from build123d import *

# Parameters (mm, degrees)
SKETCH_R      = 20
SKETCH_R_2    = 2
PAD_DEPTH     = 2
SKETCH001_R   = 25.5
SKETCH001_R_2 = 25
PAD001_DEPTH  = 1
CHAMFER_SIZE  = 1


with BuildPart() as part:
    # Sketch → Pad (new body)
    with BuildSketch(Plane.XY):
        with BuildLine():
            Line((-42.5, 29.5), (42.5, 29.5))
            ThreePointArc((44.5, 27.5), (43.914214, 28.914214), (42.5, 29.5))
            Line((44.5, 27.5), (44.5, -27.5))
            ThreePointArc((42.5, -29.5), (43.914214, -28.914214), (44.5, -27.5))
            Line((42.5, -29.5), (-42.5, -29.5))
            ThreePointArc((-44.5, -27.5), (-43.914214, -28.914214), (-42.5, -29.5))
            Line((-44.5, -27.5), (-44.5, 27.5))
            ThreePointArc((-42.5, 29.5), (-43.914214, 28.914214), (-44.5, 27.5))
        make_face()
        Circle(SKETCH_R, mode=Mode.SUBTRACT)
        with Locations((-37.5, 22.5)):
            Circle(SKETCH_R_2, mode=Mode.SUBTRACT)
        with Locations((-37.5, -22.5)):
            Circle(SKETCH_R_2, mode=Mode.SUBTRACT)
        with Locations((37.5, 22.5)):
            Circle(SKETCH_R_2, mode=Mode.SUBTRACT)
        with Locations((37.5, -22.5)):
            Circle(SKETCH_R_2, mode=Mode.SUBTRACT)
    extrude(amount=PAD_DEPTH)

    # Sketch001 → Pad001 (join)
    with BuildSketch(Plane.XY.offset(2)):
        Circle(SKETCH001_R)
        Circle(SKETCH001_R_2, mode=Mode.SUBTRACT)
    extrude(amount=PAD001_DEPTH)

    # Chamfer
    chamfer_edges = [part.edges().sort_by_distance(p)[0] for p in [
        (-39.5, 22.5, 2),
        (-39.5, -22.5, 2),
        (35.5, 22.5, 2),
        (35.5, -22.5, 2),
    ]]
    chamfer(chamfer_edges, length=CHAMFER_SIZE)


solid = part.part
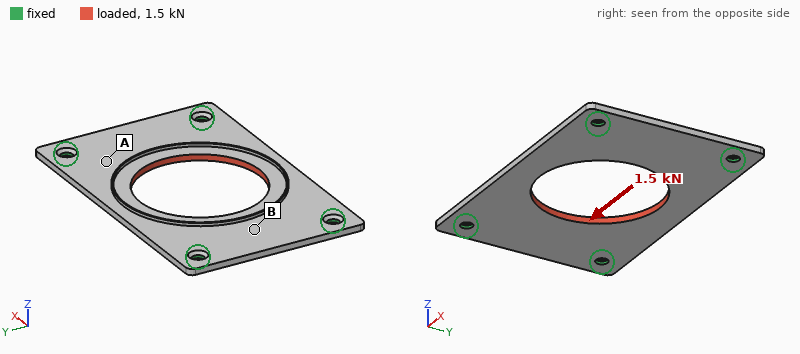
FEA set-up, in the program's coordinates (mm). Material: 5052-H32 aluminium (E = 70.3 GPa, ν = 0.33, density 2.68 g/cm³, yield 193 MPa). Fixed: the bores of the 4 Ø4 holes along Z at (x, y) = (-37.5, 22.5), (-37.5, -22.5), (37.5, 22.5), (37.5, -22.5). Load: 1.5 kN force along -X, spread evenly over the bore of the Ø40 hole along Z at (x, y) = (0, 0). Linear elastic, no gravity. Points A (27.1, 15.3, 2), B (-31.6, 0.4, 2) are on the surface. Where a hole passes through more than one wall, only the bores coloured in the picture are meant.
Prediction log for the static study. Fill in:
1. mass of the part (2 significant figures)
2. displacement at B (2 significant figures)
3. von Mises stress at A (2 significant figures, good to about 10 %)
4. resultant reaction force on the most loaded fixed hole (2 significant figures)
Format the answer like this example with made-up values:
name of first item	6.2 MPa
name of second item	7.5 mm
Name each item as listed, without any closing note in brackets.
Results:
mass of the part	21 g
displacement at B	5.4 µm
von Mises stress at A	8.1 MPa
resultant reaction force on the most loaded fixed hole	390 N
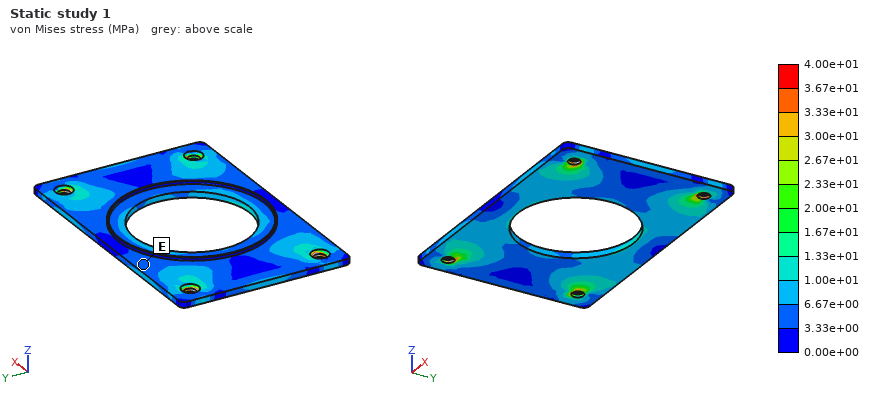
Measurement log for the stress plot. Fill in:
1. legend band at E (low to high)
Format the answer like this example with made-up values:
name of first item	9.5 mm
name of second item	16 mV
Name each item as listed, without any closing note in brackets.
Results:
legend band at E	3.33e+00 to 6.67e+00 MPa
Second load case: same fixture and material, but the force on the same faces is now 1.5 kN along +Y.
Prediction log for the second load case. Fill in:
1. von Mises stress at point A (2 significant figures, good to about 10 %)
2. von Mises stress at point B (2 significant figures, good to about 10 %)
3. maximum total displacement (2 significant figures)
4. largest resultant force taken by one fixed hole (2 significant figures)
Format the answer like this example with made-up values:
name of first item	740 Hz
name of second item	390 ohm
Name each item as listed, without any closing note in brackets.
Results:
von Mises stress at point A	11 MPa
von Mises stress at point B	16 MPa
maximum total displacement	17 µm
largest resultant force taken by one fixed hole	420 N
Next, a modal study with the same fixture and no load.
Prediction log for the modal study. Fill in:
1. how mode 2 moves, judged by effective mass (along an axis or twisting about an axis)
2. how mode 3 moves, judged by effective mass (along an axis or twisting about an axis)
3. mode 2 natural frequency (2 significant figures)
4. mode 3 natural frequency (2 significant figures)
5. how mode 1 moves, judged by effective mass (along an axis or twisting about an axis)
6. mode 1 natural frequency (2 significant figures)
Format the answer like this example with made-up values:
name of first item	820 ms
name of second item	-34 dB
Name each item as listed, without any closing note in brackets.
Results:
how mode 2 moves, judged by effective mass	twisting about X
how mode 3 moves, judged by effective mass	twisting about Y
mode 2 natural frequency	2300 Hz
mode 3 natural frequency	3700 Hz
how mode 1 moves, judged by effective mass	along Z
mode 1 natural frequency	1900 Hz
